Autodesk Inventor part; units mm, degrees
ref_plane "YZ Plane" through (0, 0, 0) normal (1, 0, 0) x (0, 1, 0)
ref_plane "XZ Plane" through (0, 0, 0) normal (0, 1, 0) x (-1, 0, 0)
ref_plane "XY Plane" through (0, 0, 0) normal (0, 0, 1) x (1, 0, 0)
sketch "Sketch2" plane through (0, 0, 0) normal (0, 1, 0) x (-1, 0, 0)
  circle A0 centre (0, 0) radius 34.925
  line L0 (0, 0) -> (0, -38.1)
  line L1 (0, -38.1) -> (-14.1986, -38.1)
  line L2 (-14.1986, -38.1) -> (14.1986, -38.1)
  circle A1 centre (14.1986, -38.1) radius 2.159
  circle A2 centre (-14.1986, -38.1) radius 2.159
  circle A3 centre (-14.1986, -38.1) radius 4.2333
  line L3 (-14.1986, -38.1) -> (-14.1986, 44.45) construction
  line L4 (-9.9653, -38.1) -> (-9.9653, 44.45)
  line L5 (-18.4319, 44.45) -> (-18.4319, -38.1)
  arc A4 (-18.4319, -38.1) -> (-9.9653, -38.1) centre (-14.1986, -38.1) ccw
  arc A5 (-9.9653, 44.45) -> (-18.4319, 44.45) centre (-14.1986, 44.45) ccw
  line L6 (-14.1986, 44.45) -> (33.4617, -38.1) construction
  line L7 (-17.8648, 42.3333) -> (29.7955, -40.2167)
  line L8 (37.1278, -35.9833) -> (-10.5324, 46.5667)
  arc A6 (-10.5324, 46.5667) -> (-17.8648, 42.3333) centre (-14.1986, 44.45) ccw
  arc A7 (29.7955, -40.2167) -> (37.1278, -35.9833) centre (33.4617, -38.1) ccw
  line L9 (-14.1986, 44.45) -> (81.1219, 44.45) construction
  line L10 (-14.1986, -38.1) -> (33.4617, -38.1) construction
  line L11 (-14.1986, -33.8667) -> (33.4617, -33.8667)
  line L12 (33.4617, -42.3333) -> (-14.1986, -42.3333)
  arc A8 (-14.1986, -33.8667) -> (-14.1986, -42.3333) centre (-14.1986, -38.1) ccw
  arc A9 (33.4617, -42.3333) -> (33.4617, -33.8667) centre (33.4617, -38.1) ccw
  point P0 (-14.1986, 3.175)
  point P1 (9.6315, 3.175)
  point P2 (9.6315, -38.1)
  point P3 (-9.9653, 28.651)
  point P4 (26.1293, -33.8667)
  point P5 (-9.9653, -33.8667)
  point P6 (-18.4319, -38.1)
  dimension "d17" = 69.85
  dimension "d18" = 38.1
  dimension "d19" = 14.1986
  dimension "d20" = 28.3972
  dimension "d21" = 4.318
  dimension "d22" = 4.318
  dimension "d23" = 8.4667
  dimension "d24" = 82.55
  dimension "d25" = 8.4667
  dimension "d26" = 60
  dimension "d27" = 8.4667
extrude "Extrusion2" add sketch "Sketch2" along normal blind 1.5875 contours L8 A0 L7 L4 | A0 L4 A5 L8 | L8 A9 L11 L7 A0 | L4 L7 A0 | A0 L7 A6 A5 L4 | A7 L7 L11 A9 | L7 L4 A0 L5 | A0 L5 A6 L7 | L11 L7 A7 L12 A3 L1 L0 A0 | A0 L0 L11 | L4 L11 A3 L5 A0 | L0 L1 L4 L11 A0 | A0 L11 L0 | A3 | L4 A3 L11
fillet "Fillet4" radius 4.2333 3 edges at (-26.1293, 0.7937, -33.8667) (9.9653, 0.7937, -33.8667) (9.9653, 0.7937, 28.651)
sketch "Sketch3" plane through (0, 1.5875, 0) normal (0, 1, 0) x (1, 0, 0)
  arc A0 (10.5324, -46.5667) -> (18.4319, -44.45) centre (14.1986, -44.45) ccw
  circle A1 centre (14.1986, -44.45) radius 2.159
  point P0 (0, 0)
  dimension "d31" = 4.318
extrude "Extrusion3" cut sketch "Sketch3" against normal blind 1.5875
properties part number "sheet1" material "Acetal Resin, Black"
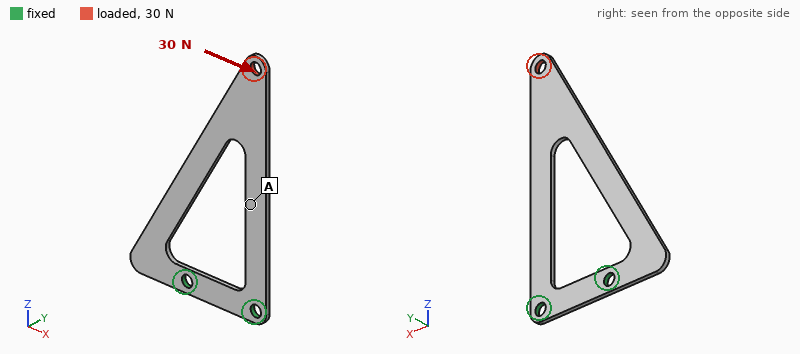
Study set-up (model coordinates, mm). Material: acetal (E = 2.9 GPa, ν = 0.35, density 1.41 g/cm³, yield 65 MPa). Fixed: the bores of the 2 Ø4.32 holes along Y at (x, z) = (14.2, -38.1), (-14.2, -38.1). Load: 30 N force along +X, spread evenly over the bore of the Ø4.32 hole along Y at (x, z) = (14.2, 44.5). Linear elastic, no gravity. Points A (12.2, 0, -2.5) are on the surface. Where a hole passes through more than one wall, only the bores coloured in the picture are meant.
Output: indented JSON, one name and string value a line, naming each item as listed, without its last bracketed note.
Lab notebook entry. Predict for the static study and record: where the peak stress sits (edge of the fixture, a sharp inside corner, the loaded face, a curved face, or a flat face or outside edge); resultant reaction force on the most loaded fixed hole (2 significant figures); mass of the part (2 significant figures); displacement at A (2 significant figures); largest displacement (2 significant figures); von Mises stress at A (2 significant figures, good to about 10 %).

{
  "where the peak stress sits": "edge of the fixture",
  "resultant reaction force on the most loaded fixed hole": "65 N",
  "mass of the part": "4.2 g",
  "displacement at A": "0.37 mm",
  "largest displacement": "1.2 mm",
  "von Mises stress at A": "3.7 MPa"
}
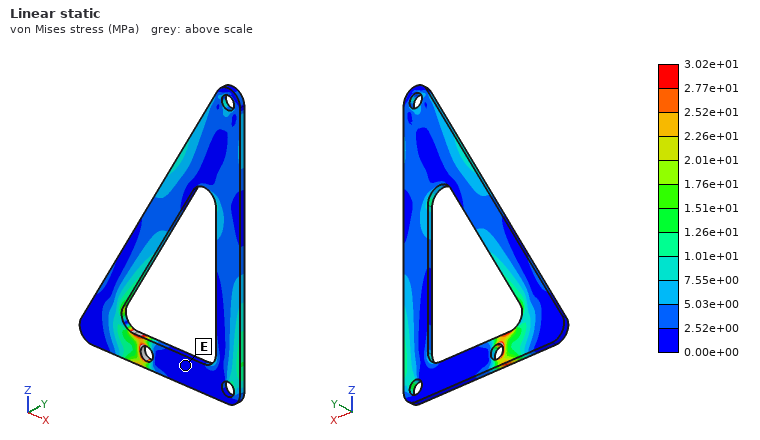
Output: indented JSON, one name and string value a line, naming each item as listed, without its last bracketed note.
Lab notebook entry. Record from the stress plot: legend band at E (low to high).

{
  "legend band at E": "0.00e+00 to 2.52e+00 MPa"
}
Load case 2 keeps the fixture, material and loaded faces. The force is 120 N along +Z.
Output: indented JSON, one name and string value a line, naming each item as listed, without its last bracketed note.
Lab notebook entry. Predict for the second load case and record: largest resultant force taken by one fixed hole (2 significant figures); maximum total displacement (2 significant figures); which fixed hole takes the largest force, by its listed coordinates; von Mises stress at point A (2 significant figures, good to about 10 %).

{
  "largest resultant force taken by one fixed hole": "120 N",
  "maximum total displacement": "0.52 mm",
  "which fixed hole takes the largest force, by its listed coordinates": "(14.2, -38.1)",
  "von Mises stress at point A": "8.6 MPa"
}
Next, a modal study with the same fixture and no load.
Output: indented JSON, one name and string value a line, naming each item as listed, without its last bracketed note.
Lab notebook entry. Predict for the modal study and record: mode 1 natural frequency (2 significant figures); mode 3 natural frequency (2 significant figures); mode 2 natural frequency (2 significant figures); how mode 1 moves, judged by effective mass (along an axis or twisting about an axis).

{
  "mode 1 natural frequency": "54 Hz",
  "mode 3 natural frequency": "380 Hz",
  "mode 2 natural frequency": "270 Hz",
  "how mode 1 moves, judged by effective mass": "along Y"
}
